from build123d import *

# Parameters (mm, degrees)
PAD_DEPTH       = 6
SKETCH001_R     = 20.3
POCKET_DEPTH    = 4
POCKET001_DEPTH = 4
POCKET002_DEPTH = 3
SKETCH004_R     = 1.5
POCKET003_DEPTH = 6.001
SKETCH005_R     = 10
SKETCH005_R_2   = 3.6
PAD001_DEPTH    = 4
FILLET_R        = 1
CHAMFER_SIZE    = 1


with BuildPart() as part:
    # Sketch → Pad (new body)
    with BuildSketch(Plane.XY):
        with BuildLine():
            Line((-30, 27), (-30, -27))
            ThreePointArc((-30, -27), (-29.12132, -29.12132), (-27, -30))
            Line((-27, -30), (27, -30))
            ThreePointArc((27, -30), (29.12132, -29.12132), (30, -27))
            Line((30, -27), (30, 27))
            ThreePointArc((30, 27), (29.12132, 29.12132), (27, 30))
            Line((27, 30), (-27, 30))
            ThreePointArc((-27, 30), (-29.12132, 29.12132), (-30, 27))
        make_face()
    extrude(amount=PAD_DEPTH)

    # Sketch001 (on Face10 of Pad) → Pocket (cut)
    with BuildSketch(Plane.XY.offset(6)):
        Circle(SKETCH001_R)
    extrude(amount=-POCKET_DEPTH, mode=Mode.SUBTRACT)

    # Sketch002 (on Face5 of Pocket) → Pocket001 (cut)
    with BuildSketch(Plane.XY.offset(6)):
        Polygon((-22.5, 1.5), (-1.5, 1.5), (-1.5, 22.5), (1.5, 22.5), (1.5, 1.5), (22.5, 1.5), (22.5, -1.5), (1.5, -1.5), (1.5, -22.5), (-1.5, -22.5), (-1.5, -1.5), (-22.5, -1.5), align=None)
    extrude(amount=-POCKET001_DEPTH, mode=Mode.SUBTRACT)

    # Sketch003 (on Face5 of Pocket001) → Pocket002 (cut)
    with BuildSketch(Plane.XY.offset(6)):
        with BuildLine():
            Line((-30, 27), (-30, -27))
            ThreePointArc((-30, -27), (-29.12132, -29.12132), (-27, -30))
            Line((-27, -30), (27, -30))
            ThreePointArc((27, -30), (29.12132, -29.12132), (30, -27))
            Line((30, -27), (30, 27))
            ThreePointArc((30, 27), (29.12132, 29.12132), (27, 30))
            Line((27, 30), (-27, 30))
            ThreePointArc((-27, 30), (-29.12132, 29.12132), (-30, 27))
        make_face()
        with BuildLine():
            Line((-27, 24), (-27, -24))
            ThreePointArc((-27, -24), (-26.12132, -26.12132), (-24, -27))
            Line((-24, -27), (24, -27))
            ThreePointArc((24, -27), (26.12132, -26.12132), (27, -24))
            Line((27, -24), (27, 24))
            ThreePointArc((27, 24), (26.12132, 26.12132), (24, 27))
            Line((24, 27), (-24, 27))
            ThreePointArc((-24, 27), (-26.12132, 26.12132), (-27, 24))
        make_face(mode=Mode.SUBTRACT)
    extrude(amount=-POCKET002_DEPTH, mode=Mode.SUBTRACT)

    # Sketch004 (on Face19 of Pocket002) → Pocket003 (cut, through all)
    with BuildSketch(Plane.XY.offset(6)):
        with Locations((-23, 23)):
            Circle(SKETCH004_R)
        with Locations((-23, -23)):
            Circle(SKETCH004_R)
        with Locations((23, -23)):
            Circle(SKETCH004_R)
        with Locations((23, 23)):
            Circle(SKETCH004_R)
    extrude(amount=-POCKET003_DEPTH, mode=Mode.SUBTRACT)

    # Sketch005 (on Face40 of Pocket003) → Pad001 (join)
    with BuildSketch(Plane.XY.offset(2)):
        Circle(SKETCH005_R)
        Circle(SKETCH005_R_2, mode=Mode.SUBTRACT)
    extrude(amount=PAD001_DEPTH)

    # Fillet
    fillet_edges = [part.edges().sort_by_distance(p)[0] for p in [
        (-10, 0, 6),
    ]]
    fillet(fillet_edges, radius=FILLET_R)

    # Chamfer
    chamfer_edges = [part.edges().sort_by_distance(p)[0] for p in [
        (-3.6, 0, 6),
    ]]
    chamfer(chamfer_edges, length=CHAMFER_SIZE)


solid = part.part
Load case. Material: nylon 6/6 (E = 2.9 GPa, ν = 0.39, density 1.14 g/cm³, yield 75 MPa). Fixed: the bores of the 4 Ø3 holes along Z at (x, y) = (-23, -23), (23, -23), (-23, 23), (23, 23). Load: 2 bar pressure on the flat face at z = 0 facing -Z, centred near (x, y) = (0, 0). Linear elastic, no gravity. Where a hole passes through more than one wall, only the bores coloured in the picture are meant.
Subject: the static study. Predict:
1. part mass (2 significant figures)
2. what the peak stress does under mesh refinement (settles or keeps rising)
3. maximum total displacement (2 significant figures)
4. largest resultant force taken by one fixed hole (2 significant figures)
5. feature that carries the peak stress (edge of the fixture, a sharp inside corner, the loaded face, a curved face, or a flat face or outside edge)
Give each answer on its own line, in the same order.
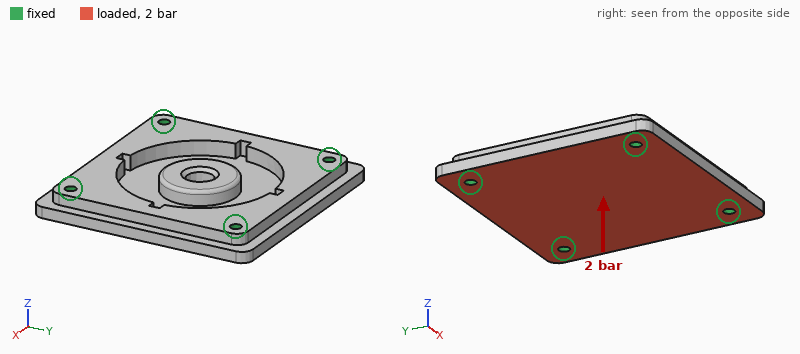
17 g
keeps rising
0.29 mm
200 N
edge of the fixture
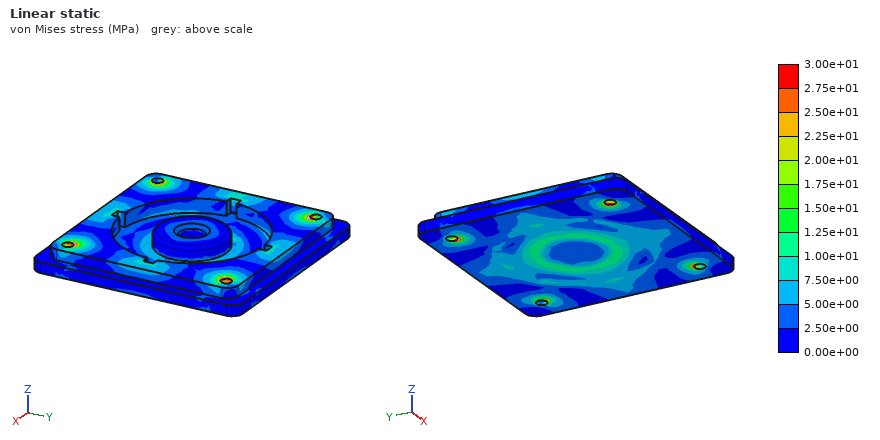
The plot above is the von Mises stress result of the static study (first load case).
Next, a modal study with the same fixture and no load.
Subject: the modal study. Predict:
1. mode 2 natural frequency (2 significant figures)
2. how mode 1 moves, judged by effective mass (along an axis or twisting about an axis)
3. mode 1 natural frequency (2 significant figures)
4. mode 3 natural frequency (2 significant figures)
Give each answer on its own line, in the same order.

3800 Hz
along Z
2500 Hz
3800 Hz
